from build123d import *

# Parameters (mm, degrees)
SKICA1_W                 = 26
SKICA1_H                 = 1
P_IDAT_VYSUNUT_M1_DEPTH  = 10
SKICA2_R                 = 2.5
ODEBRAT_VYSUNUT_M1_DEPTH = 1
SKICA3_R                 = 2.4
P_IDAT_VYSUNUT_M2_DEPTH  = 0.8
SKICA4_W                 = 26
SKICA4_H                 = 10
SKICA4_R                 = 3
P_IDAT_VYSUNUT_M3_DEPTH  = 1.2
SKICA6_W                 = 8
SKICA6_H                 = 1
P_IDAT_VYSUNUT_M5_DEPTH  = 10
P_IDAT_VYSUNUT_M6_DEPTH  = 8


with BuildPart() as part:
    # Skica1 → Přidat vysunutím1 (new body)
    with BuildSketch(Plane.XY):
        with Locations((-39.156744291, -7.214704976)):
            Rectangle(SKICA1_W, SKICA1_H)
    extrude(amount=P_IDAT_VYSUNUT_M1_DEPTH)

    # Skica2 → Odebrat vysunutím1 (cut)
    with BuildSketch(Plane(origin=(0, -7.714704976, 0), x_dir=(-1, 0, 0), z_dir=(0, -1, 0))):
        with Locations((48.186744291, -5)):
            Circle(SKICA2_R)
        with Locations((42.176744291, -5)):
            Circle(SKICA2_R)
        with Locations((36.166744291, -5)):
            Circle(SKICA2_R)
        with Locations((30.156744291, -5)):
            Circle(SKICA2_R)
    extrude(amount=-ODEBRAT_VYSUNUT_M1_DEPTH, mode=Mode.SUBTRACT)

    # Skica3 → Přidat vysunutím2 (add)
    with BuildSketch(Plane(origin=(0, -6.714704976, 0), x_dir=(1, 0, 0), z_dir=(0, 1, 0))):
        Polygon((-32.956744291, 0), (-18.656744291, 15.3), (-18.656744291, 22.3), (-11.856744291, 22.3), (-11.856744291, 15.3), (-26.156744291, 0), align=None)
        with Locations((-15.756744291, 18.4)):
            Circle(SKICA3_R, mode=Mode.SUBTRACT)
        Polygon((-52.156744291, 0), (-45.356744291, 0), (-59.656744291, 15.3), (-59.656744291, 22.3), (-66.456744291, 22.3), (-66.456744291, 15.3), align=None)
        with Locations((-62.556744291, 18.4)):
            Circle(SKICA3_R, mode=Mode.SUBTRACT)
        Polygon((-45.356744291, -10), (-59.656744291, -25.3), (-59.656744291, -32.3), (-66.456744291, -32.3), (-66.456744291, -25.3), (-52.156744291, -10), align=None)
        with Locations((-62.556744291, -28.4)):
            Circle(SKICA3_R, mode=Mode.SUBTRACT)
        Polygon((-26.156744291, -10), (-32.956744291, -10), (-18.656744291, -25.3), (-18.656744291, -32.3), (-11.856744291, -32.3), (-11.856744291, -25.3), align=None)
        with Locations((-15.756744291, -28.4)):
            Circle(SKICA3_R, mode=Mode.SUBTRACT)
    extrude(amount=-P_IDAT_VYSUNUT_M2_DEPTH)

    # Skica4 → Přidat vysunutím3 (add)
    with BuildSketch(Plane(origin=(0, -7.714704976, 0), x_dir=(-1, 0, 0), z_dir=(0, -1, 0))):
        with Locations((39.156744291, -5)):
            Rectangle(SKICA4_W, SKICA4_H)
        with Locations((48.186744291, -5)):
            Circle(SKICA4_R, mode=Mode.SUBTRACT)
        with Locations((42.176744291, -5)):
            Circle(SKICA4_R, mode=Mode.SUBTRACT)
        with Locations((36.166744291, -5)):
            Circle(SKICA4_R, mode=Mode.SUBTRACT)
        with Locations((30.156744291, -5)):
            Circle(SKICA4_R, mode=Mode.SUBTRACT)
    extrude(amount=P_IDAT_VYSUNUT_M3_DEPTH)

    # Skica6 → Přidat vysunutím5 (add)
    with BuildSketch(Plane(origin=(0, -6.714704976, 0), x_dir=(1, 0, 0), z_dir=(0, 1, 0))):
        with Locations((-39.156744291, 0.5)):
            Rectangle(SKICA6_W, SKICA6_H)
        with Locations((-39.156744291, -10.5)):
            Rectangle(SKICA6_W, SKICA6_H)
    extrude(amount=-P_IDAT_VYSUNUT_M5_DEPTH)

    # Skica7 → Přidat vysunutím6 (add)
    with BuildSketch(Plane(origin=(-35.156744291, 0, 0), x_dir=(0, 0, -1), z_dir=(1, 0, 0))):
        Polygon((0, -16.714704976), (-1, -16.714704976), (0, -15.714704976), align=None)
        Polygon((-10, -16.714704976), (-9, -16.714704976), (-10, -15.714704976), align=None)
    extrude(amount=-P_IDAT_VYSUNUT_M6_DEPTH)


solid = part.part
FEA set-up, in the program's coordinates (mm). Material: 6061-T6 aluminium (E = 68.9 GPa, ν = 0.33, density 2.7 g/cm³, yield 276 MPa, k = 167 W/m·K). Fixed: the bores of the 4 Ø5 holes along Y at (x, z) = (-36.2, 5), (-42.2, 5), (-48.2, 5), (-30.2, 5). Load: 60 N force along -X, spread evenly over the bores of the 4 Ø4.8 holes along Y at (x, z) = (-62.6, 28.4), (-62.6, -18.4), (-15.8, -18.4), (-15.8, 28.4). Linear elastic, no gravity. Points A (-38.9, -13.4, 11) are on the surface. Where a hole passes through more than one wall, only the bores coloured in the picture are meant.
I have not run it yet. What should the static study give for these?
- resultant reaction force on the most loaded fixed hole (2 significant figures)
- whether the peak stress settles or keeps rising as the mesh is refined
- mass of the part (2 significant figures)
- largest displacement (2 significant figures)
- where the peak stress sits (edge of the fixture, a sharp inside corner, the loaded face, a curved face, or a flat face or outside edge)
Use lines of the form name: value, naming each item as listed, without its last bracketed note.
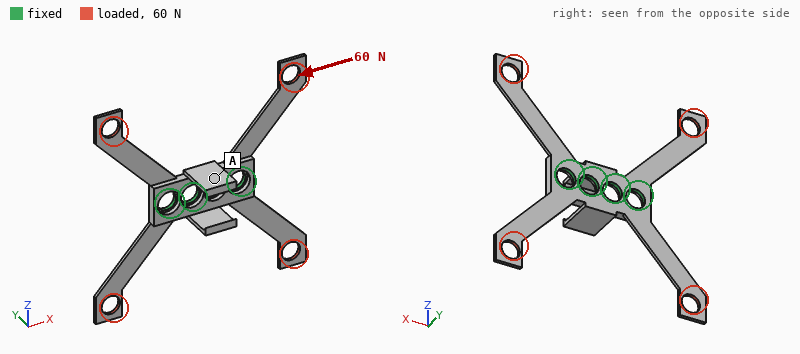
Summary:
resultant reaction force on the most loaded fixed hole: 57 N
whether the peak stress settles or keeps rising as the mesh is refined: keeps rising
mass of the part: 2.6 g
largest displacement: 0.14 mm
where the peak stress sits: a sharp inside corner
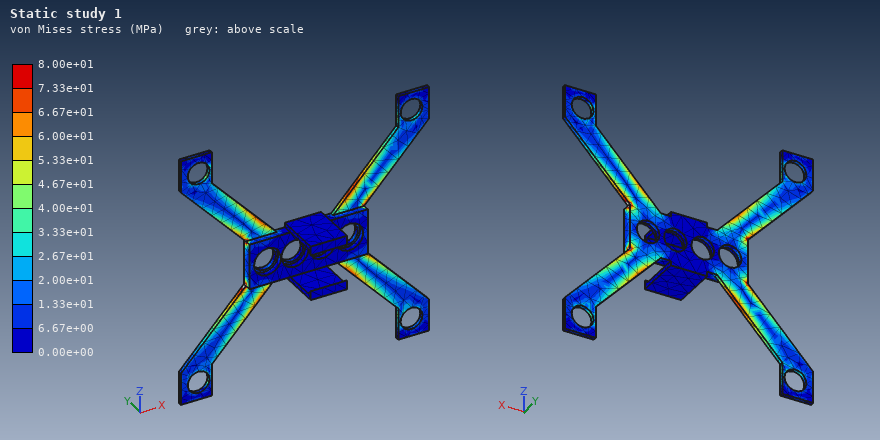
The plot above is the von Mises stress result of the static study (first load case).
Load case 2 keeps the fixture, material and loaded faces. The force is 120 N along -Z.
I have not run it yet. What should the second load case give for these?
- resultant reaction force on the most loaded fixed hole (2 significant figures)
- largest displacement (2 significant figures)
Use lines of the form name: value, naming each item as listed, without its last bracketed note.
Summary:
resultant reaction force on the most loaded fixed hole: 120 N
largest displacement: 0.17 mm
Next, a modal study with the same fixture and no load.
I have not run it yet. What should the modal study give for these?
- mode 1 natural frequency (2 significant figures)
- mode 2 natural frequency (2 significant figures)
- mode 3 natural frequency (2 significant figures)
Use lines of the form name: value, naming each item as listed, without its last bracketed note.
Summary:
mode 1 natural frequency: 930 Hz
mode 2 natural frequency: 930 Hz
mode 3 natural frequency: 940 Hz
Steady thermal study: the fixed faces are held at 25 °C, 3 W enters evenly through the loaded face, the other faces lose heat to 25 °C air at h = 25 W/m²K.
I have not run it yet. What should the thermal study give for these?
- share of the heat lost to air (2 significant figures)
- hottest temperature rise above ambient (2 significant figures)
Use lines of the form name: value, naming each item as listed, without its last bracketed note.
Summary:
share of the heat lost to air: 15 %
hottest temperature rise above ambient: 28 K
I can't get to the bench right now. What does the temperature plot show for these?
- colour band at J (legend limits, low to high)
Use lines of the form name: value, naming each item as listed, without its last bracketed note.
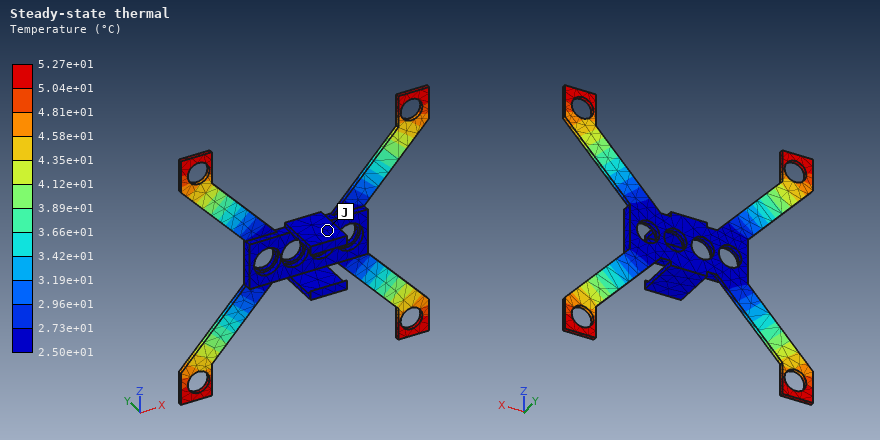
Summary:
colour band at J: 2.50e+01 to 2.73e+01 °C
